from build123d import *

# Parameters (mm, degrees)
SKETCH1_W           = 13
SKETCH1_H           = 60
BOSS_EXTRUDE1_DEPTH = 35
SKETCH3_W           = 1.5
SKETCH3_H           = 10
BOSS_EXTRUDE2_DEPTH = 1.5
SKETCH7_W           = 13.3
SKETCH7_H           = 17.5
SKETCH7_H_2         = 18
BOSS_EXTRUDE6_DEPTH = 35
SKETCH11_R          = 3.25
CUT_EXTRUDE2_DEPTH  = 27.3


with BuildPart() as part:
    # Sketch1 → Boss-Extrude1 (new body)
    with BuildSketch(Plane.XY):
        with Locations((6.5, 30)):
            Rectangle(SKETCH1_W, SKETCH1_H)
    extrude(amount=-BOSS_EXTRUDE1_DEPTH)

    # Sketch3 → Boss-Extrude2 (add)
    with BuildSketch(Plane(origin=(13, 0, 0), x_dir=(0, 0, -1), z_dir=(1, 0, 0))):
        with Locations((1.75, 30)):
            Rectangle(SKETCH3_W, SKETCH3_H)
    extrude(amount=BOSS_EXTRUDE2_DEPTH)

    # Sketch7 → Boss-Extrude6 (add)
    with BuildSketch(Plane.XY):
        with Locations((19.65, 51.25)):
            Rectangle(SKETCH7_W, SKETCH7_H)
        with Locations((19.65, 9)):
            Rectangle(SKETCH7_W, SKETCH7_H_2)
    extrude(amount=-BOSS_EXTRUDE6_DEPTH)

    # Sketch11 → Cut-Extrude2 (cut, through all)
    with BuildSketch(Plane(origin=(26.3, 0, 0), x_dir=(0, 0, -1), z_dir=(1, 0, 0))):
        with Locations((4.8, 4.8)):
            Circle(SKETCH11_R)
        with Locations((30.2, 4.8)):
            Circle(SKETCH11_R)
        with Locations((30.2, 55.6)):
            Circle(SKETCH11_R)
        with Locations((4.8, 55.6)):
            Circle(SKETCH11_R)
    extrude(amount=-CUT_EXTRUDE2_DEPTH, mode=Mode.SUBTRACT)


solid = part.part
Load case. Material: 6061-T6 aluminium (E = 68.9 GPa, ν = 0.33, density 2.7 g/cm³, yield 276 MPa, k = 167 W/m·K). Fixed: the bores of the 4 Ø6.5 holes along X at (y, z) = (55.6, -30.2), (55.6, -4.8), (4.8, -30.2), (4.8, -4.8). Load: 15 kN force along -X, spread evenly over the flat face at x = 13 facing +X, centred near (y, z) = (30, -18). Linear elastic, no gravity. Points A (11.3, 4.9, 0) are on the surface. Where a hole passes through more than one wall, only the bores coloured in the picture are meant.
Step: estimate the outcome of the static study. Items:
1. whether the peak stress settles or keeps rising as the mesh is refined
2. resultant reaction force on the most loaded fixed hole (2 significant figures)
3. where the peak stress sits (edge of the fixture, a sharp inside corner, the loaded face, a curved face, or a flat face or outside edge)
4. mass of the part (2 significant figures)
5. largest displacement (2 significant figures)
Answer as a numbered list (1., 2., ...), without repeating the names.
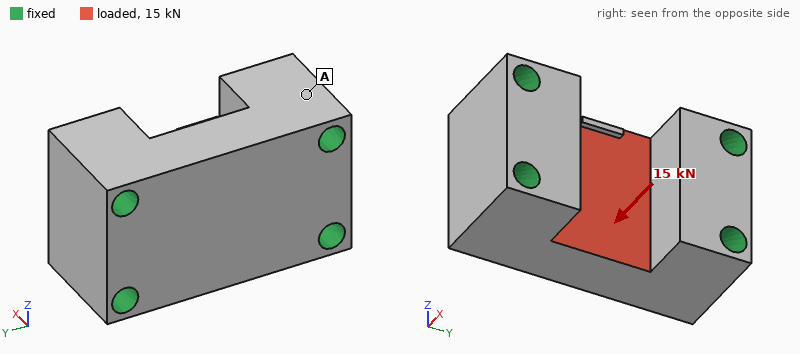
1. keeps rising
2. 3.9 kN
3. edge of the fixture
4. 110 g
5. 19 µm
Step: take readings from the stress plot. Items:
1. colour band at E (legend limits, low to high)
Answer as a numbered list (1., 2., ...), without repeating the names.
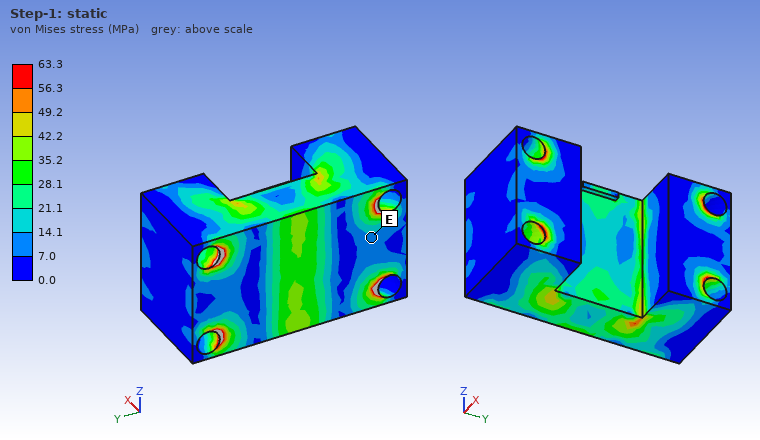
1. 7.0 to 14.1 MPa
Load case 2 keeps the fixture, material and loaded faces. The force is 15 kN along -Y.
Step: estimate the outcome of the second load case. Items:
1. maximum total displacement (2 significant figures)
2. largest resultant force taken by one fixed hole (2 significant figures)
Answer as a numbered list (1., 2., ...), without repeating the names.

1. 8.1 µm
2. 4.0 kN
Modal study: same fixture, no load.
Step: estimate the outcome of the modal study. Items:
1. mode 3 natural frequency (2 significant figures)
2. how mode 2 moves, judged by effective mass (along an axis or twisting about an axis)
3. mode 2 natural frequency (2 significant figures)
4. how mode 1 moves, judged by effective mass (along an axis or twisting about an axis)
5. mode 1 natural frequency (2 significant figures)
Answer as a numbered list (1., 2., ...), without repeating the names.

1. 35 kHz
2. along Z
3. 31 kHz
4. along X
5. 28 kHz
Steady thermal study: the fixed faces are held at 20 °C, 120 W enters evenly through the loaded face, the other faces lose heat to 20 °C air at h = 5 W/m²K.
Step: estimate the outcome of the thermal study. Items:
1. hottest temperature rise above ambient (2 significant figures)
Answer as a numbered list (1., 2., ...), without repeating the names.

1. 15 K
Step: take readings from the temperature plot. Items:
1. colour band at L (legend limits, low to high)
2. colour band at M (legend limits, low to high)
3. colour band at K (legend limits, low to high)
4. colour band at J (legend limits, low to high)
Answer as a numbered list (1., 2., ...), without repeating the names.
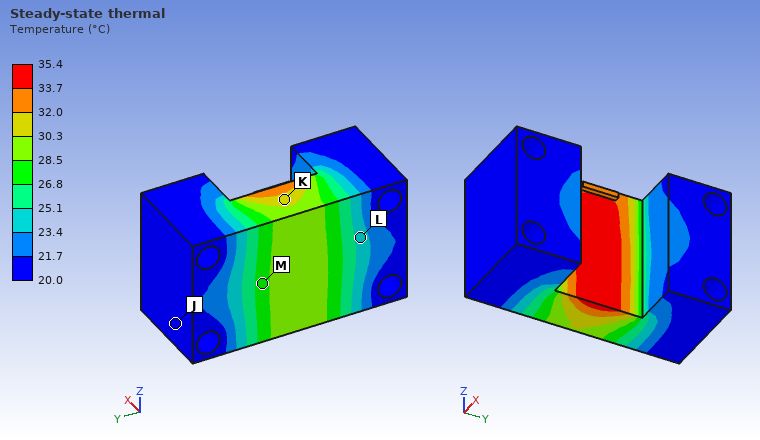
1. 23.4 to 25.1 °C
2. 26.8 to 28.5 °C
3. 30.3 to 32.0 °C
4. 20.0 to 21.7 °C
